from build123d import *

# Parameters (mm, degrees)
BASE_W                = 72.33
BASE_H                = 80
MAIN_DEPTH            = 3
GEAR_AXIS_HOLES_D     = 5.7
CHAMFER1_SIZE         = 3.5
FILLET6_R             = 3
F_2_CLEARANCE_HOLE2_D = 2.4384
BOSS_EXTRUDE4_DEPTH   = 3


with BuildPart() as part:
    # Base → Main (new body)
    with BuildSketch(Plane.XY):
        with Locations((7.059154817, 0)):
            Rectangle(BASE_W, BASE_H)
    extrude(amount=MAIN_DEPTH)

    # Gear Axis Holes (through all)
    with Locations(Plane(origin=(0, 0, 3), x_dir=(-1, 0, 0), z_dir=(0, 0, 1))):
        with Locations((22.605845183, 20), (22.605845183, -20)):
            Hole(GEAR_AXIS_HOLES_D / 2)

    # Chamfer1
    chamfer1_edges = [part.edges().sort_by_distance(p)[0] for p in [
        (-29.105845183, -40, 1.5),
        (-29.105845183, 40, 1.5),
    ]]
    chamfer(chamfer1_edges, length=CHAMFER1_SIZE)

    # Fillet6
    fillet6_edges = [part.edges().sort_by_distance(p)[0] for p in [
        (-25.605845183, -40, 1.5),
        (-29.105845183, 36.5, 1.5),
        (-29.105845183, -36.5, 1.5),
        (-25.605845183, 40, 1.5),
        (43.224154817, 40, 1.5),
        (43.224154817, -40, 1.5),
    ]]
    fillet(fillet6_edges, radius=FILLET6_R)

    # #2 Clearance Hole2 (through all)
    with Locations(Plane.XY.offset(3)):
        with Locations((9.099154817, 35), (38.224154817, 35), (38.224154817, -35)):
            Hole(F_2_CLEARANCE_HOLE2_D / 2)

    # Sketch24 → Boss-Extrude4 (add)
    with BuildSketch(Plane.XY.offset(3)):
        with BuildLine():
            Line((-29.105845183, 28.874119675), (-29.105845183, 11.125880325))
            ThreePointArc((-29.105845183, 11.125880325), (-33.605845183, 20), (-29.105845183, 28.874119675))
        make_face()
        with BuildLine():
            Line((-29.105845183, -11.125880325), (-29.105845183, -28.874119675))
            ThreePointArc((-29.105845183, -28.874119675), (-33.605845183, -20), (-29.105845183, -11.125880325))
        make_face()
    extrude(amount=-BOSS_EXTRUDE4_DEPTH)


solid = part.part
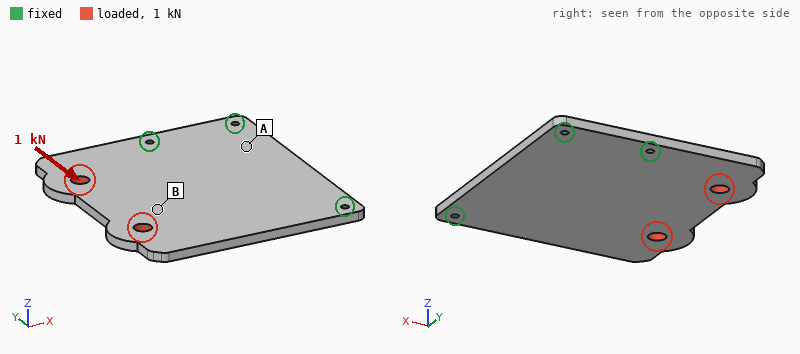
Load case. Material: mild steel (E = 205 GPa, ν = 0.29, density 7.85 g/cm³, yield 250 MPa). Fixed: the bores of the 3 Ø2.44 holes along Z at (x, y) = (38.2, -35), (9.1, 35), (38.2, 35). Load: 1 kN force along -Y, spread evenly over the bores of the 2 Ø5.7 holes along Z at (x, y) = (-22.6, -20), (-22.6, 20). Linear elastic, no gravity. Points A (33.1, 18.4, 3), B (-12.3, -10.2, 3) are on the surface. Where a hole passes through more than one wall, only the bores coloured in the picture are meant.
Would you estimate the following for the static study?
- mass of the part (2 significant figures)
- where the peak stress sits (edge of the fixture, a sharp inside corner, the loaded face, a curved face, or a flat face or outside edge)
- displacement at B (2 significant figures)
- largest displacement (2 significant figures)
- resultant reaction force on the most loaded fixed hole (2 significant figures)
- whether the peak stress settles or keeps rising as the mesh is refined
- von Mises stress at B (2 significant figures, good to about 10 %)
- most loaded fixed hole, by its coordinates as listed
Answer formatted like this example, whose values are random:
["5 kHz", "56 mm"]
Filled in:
["140 g", "edge of the fixture", "3.5 µm", "5.7 µm", "820 N", "keeps rising", "8.8 MPa", "(9.1, 35)"]
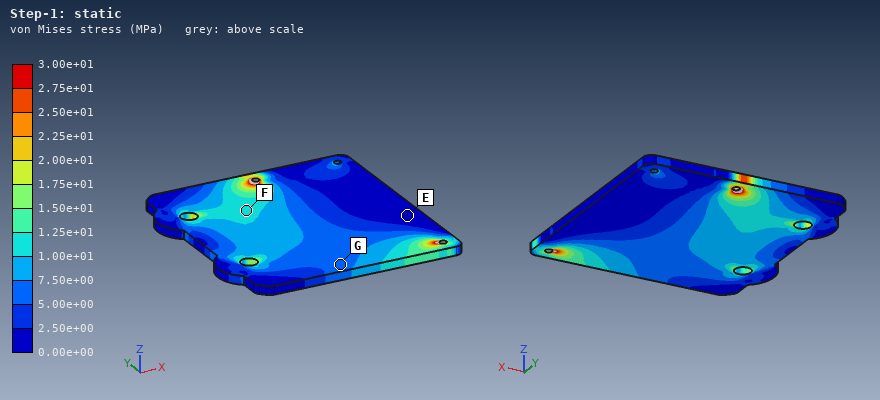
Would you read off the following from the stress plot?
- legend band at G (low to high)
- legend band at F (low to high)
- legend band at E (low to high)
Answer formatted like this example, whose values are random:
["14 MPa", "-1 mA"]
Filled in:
["5.00e+00 to 7.50e+00 MPa", "1.00e+01 to 1.25e+01 MPa", "0.00e+00 to 2.50e+00 MPa"]
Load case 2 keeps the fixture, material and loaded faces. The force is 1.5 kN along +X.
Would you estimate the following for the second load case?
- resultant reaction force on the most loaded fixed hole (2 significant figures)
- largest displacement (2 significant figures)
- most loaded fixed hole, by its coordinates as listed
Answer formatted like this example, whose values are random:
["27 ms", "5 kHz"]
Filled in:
["740 N", "4.1 µm", "(38.2, -35)"]
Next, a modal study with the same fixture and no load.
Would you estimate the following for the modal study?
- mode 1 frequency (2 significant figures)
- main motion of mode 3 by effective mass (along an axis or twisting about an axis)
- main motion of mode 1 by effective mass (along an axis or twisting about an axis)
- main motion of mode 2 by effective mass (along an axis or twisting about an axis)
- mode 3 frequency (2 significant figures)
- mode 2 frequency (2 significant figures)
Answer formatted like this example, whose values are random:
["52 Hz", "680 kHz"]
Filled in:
["680 Hz", "along Z", "along Z", "twisting about X", "2700 Hz", "1800 Hz"]
